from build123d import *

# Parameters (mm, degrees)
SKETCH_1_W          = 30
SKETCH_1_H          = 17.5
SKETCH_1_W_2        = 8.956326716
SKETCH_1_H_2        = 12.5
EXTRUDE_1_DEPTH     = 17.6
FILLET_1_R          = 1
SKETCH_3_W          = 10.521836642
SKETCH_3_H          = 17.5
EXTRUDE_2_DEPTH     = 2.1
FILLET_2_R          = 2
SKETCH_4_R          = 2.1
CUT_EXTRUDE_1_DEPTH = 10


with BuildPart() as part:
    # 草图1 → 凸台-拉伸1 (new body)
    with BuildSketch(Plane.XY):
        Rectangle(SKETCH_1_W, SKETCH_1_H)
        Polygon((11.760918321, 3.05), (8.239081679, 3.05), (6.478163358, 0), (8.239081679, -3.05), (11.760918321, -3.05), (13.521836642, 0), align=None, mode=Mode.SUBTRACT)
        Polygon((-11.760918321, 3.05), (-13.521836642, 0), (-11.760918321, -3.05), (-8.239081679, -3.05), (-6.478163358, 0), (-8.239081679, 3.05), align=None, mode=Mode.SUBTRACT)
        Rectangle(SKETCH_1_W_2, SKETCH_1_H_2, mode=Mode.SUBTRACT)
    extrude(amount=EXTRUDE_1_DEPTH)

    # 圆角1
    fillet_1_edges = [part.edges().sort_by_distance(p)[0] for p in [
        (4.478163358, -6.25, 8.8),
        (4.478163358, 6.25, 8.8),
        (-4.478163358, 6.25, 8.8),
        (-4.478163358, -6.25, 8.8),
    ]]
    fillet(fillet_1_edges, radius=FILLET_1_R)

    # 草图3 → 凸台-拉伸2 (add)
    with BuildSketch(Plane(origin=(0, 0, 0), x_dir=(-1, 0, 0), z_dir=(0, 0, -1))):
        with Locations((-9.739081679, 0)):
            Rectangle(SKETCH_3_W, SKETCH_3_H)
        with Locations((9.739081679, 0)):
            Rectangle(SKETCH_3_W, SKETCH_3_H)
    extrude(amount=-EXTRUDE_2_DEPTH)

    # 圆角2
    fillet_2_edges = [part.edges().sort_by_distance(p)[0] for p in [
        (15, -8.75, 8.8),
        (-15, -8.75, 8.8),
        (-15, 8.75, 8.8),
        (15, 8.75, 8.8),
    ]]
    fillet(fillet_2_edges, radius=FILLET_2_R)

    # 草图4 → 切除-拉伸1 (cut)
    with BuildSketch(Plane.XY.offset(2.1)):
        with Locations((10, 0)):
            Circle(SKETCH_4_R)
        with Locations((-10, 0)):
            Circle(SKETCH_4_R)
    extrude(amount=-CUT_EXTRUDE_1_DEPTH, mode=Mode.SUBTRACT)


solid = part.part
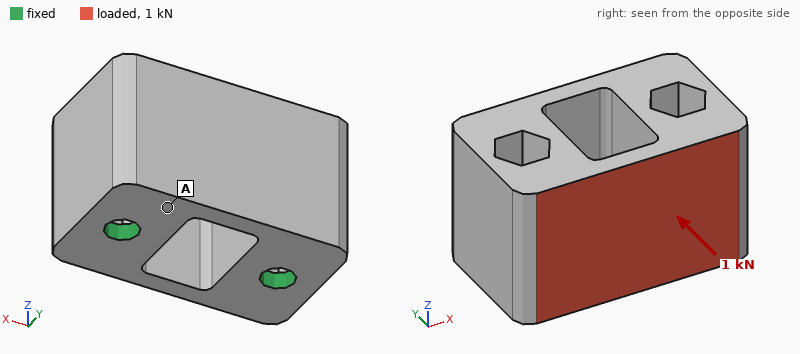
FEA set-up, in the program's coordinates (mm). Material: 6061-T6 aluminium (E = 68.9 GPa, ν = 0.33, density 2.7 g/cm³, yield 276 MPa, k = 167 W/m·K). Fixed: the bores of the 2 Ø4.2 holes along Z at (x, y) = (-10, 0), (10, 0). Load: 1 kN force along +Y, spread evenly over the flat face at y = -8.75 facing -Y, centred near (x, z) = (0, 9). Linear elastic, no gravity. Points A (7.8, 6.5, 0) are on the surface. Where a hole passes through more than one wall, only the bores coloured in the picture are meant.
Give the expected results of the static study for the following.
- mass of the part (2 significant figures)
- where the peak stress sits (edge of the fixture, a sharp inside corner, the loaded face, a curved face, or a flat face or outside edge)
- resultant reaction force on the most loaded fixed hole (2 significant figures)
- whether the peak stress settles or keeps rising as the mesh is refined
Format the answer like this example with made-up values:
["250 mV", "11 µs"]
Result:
["17 g", "edge of the fixture", "500 N", "keeps rising"]
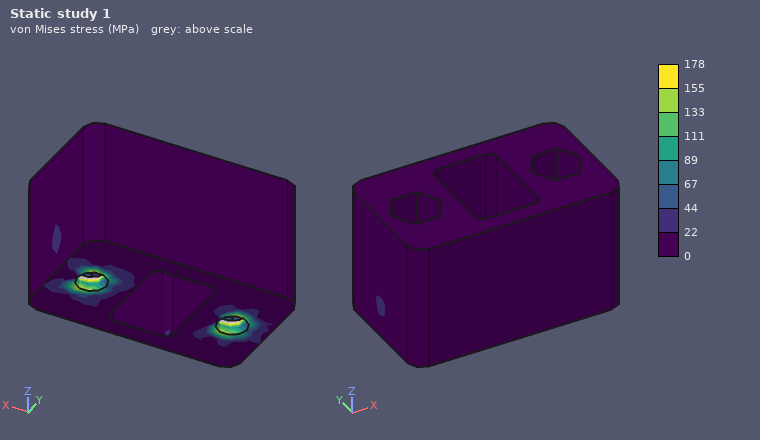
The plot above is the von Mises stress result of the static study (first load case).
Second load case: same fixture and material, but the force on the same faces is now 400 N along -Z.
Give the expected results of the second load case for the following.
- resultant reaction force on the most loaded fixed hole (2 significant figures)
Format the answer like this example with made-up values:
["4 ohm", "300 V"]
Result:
["200 N"]
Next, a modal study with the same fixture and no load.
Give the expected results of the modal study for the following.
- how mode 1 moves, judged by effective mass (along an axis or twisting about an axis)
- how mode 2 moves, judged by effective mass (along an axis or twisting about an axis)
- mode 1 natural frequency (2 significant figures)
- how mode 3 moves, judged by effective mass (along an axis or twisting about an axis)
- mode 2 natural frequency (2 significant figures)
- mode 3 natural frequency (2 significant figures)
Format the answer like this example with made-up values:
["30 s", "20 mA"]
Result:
["along Y", "along X", "6500 Hz", "twisting about Z", "17 kHz", "18 kHz"]
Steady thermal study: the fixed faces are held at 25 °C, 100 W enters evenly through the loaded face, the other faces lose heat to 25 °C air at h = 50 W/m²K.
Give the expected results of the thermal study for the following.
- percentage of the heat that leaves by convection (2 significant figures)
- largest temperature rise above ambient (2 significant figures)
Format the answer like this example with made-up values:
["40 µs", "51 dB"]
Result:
["4.1 %", "50 K"]
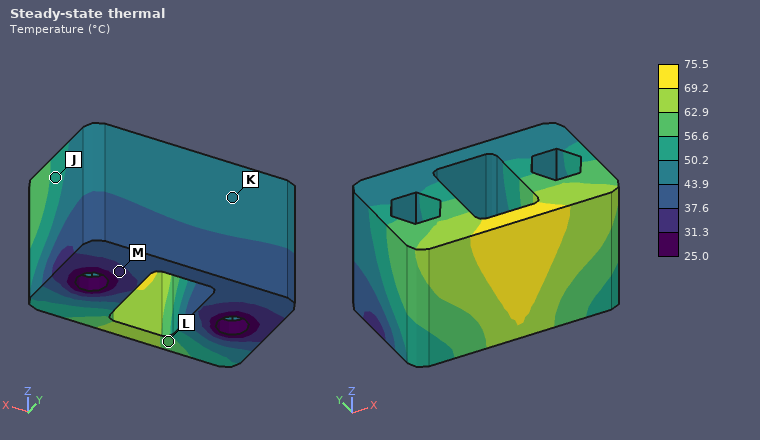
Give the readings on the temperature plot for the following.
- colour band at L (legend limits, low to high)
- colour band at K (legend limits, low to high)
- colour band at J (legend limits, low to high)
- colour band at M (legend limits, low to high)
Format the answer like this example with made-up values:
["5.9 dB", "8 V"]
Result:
["56.6 to 62.9 °C", "43.9 to 50.2 °C", "50.2 to 56.6 °C", "31.3 to 37.6 °C"]
